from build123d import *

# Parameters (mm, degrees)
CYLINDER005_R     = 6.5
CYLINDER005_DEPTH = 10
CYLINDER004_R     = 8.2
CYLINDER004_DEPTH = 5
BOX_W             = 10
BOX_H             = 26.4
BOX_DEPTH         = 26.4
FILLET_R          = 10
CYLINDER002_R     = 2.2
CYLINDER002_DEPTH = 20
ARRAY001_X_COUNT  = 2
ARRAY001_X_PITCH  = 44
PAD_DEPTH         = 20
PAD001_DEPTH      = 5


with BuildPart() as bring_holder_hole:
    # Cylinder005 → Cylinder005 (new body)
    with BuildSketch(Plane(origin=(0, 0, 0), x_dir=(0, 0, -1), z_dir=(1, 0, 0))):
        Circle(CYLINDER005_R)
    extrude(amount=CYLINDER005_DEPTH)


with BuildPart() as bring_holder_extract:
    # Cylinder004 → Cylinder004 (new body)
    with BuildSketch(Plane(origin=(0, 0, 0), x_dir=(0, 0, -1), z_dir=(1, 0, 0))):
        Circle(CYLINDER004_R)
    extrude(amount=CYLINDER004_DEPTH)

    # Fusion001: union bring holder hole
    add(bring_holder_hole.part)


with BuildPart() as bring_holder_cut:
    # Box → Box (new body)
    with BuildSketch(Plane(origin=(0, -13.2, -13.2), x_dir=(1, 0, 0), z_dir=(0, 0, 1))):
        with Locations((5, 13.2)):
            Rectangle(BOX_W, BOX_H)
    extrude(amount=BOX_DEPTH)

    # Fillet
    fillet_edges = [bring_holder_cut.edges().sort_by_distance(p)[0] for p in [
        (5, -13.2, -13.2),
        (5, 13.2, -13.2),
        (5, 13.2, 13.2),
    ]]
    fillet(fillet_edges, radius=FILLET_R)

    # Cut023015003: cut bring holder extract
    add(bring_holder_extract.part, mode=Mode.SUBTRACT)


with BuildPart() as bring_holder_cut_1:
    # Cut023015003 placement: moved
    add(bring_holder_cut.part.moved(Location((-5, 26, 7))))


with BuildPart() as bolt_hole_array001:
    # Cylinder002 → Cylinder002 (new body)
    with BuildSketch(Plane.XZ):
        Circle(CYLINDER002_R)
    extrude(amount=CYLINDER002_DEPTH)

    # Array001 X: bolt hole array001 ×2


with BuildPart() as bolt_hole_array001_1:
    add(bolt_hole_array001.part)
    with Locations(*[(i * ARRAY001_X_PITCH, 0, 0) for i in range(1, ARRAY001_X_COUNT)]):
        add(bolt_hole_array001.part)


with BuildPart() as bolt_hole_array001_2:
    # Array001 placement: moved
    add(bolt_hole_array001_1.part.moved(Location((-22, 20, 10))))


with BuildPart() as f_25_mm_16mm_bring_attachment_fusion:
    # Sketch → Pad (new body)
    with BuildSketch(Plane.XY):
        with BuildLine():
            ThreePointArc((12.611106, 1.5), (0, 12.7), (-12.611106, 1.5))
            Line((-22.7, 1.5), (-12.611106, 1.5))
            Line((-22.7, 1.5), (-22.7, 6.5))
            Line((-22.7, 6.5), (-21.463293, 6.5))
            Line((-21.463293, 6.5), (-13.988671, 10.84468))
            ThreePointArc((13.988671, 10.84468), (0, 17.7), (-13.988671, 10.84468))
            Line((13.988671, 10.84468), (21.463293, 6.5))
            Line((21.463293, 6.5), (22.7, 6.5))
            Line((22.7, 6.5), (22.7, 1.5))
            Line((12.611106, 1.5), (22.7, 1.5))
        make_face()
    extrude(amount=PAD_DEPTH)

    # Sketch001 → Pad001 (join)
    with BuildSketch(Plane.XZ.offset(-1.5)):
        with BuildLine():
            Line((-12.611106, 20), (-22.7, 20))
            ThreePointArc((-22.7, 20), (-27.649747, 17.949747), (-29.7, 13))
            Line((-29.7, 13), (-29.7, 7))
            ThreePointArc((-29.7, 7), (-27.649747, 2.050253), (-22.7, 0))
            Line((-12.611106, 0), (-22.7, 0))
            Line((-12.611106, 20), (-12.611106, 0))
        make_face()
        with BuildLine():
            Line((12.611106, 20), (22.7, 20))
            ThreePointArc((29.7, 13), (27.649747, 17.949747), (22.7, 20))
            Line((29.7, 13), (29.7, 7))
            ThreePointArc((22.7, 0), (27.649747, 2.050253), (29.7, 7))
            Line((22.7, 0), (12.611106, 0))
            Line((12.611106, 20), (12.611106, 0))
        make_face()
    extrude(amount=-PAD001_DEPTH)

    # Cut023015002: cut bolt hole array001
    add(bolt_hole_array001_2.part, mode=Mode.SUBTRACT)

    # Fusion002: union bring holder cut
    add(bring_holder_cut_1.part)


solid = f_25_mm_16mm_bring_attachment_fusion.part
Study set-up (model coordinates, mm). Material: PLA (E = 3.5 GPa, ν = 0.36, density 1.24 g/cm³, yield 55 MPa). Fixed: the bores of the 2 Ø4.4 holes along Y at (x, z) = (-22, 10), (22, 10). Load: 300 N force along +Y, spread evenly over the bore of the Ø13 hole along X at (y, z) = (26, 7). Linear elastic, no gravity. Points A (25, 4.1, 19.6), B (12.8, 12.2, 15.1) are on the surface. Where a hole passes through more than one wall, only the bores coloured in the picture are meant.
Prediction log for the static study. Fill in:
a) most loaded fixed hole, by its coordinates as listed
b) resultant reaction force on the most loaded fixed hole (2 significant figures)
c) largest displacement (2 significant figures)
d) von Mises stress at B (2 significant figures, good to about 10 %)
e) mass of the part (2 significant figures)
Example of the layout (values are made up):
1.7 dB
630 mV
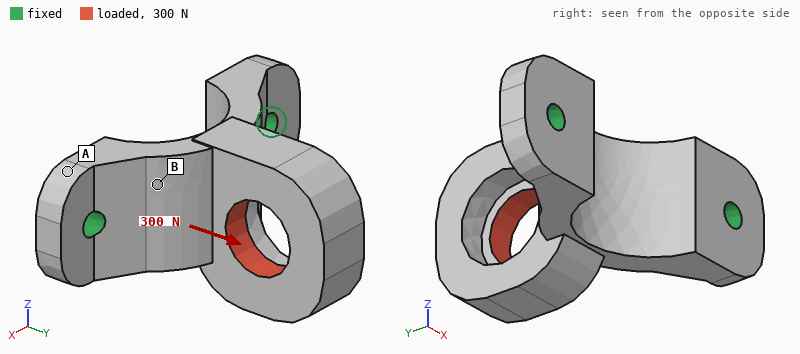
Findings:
(22, 10)
260 N
0.18 mm
3.3 MPa
13 g
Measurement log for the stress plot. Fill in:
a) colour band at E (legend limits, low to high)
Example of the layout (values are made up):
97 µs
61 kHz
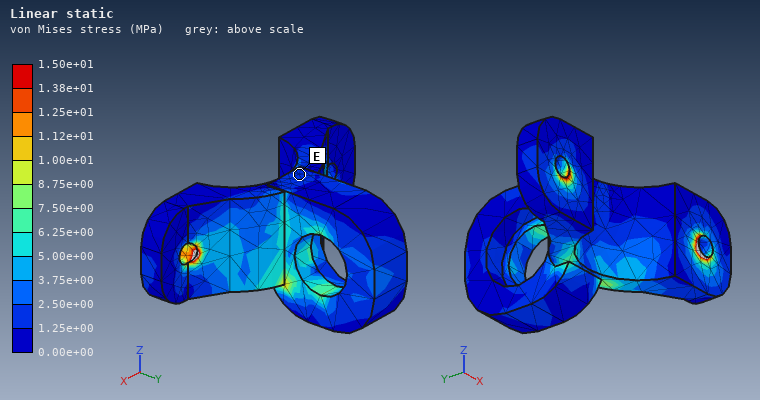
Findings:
1.25e+00 to 2.50e+00 MPa
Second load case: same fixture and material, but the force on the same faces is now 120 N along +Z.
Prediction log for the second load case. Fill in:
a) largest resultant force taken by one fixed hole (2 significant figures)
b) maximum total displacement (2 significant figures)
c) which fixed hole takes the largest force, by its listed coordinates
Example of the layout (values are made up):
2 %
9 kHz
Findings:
67 N
0.37 mm
(22, 10)
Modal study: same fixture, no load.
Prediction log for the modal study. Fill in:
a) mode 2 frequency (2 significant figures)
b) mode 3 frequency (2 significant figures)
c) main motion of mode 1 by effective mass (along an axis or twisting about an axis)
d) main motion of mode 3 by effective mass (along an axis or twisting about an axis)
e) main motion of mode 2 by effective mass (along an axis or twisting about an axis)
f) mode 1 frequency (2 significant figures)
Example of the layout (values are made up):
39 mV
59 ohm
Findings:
2400 Hz
4900 Hz
along Z
along Y
along X
1300 Hz
